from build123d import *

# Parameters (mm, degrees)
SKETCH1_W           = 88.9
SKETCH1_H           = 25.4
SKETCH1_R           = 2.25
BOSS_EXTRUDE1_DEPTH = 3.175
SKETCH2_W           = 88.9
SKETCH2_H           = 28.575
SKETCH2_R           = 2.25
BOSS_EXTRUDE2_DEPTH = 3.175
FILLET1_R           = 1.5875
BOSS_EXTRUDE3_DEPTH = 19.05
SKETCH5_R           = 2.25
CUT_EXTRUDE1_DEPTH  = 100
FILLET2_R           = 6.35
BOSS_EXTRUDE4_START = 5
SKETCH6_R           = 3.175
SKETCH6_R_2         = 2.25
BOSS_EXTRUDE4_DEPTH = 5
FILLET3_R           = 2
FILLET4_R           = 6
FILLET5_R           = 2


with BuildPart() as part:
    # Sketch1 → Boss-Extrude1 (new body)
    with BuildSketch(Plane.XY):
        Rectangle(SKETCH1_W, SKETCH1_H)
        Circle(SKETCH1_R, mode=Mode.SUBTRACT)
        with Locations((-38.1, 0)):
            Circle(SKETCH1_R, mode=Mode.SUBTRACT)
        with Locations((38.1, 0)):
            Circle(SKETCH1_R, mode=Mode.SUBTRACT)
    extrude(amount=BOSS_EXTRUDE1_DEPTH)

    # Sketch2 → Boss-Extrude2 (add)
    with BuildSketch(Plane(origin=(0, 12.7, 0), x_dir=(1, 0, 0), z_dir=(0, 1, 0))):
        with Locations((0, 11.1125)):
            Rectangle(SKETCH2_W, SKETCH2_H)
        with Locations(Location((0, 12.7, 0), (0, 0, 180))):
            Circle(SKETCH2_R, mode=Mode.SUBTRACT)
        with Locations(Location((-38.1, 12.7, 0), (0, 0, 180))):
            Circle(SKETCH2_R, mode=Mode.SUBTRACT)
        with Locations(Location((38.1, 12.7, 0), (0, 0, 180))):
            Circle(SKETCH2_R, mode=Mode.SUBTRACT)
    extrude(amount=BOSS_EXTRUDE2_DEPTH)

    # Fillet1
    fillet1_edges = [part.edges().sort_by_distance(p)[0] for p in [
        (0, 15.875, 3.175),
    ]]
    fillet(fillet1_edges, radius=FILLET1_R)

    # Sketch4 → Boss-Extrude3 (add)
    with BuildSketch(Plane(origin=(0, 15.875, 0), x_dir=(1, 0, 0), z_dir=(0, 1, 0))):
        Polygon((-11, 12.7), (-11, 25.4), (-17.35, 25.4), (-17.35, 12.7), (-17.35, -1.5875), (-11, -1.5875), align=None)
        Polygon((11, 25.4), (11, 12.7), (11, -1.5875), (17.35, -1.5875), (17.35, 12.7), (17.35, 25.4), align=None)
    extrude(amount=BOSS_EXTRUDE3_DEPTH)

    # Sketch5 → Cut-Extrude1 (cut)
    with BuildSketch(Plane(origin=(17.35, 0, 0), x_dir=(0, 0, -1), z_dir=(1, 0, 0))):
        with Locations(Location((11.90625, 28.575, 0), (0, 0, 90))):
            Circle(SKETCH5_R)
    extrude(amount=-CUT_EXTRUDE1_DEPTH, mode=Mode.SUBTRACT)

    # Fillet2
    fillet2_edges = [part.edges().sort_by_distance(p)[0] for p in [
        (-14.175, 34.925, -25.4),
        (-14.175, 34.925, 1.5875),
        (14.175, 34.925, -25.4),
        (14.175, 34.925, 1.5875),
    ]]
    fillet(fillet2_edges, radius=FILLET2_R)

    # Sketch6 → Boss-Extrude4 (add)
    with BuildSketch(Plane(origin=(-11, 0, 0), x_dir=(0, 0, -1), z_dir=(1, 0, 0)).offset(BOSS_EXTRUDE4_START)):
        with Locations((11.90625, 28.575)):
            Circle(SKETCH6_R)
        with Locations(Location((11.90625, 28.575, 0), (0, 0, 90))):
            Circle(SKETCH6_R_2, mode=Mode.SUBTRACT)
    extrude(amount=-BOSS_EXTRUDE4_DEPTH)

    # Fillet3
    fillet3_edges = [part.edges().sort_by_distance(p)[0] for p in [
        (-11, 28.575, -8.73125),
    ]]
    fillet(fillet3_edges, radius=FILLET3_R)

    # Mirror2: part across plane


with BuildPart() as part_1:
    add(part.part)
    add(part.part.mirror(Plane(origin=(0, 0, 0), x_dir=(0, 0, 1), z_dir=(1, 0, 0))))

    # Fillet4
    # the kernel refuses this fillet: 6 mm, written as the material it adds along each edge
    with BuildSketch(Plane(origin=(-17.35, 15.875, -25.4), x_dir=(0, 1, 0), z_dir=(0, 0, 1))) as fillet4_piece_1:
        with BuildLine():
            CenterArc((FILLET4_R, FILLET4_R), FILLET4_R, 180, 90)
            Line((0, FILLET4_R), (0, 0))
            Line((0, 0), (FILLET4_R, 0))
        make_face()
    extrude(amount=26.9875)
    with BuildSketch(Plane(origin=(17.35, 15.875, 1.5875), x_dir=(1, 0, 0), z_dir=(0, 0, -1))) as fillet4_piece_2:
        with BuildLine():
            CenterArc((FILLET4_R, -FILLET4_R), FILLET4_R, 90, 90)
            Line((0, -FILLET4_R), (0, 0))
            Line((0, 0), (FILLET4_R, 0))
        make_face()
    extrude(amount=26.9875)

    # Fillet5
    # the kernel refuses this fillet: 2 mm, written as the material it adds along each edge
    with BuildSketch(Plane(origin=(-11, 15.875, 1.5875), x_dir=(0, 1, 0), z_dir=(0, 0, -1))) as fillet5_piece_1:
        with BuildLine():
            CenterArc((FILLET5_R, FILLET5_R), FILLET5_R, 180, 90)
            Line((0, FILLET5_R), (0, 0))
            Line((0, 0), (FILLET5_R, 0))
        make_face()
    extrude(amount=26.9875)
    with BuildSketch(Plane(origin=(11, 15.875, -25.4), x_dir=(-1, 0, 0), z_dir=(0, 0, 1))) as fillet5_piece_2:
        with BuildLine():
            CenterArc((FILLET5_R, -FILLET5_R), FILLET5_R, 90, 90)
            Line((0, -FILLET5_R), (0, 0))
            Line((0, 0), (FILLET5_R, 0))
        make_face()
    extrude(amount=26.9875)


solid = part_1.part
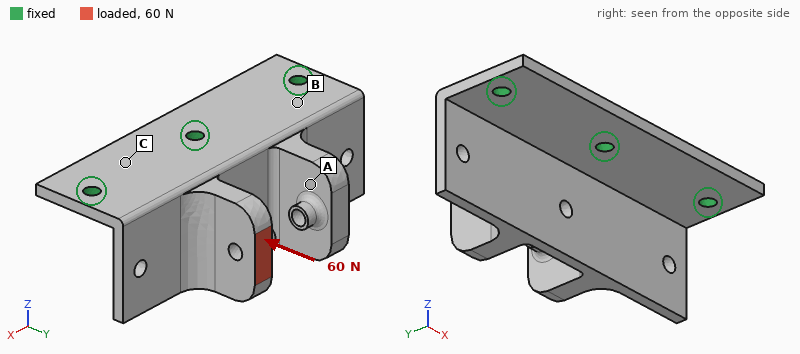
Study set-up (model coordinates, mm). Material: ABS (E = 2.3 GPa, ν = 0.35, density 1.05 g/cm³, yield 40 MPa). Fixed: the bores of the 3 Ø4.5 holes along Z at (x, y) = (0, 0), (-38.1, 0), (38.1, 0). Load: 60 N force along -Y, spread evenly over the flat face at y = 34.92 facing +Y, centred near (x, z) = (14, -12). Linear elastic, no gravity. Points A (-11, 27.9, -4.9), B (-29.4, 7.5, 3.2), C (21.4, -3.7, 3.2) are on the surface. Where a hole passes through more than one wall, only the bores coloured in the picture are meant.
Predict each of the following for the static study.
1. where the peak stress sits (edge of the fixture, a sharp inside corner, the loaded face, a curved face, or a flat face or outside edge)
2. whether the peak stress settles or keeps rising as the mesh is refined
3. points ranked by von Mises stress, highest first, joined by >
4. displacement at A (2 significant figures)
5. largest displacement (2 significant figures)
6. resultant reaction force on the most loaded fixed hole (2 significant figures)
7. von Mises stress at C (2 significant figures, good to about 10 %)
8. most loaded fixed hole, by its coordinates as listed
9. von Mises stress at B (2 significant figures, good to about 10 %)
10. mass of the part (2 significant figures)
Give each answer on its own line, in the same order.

edge of the fixture
keeps rising
B > C > A
0.45 mm
1.1 mm
46 N
1.6 MPa
(0, 0)
3.2 MPa
23 g
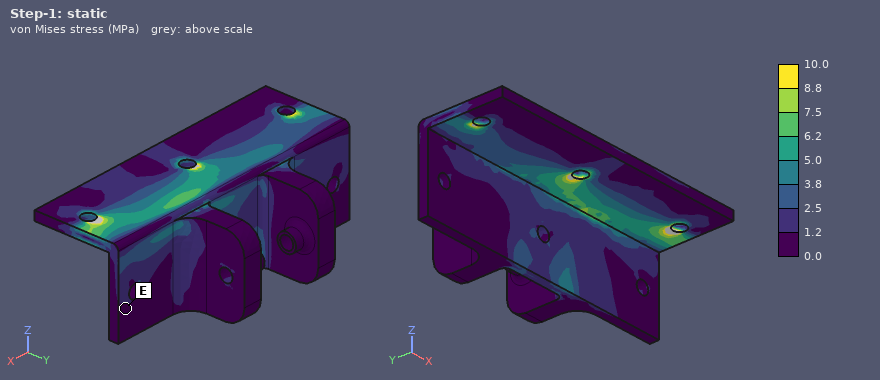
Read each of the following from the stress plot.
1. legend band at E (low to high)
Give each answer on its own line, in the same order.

0.0 to 1.2 MPa
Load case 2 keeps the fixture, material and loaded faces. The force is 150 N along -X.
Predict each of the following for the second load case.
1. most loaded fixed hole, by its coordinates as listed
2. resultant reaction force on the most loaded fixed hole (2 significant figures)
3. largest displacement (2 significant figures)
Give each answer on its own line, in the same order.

(38.1, 0)
130 N
0.75 mm
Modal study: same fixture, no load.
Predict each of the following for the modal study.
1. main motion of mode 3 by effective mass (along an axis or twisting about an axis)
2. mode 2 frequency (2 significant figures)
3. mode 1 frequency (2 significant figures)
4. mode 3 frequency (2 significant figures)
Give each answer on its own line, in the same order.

along X
800 Hz
360 Hz
1500 Hz
